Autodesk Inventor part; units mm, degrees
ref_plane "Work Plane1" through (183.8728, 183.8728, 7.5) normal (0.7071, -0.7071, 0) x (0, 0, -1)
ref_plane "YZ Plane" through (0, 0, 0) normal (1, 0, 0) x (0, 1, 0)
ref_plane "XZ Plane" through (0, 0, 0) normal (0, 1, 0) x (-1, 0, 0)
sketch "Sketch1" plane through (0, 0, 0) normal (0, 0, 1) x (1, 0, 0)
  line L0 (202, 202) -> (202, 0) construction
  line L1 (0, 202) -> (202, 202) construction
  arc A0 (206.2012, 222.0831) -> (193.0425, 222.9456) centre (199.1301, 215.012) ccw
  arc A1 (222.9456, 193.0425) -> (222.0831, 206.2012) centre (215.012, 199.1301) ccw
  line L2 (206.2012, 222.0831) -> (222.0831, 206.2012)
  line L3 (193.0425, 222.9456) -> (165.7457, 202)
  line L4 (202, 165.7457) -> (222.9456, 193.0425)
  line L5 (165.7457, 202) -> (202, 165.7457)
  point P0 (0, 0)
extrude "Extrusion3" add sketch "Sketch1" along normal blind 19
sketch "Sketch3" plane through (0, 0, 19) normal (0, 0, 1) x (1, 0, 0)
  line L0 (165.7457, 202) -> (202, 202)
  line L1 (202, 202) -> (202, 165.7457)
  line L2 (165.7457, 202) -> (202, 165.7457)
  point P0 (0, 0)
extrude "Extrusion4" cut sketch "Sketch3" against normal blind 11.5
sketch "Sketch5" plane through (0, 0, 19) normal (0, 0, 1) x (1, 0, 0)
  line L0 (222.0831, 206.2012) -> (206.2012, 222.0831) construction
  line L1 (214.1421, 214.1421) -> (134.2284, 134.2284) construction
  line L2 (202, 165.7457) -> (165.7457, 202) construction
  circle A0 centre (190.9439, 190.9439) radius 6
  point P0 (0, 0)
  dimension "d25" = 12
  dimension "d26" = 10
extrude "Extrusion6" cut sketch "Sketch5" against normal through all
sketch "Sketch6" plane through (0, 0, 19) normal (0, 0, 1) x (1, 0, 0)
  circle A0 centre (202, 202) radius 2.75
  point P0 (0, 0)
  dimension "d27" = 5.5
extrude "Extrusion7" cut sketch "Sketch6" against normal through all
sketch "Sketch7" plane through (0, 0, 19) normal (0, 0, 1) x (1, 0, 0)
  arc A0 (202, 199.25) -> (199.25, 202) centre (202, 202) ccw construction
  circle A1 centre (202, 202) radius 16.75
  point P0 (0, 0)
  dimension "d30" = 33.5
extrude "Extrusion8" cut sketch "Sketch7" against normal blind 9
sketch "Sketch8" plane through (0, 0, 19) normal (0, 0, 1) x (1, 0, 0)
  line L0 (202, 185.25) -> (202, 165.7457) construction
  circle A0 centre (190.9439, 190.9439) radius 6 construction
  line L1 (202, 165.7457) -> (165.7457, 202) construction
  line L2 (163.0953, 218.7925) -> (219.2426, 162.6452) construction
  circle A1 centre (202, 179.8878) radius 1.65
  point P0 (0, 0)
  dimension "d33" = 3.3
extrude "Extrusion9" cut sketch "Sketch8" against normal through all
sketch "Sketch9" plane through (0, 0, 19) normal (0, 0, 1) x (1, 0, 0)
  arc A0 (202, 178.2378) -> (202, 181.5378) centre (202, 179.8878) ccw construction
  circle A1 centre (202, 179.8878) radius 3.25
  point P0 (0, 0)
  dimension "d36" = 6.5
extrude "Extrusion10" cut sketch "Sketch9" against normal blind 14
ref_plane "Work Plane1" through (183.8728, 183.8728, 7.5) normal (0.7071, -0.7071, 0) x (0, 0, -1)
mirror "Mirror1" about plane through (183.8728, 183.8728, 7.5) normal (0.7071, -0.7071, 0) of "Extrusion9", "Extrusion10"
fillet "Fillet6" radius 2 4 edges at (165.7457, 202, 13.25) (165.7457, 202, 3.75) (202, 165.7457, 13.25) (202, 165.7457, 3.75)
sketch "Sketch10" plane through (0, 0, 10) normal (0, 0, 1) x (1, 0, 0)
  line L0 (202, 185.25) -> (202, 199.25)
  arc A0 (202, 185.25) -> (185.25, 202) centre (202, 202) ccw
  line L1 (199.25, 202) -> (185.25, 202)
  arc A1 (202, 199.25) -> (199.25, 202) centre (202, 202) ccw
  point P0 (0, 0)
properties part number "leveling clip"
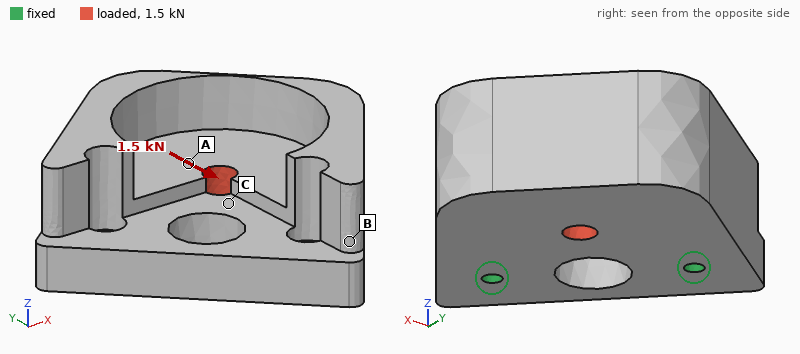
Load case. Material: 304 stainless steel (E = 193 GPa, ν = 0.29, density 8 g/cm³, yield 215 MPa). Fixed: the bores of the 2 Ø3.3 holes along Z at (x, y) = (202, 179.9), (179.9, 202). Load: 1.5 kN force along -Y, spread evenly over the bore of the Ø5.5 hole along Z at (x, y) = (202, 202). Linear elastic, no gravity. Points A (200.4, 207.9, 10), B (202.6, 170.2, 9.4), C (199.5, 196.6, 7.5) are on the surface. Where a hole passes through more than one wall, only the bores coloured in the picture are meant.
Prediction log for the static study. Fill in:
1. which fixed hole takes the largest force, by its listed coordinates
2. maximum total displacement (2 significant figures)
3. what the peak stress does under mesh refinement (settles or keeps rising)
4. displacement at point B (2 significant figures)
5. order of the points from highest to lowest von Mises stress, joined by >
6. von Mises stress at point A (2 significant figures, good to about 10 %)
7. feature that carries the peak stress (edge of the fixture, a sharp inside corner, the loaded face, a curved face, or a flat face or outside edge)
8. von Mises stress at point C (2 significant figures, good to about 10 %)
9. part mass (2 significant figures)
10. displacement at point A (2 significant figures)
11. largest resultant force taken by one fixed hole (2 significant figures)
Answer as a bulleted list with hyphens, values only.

- (202, 179.9)
- 4.0 µm
- keeps rising
- 1.7 µm
- C > A > B
- 6.3 MPa
- edge of the fixture
- 16 MPa
- 170 g
- 2.6 µm
- 1.2 kN
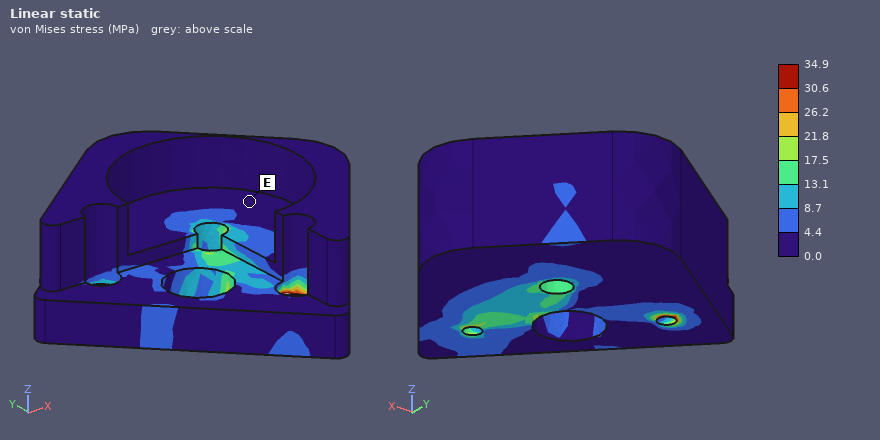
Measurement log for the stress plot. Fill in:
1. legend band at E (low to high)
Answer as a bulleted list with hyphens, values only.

- 0.0 to 4.4 MPa
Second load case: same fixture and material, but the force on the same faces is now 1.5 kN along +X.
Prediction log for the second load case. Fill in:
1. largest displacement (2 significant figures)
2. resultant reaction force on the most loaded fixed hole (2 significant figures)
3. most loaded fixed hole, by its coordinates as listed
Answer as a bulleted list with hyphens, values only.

- 4.0 µm
- 1.2 kN
- (179.9, 202)
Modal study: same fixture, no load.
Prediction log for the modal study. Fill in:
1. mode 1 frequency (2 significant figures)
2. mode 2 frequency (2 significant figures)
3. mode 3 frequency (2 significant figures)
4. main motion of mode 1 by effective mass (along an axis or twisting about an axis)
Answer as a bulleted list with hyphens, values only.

- 3200 Hz
- 7700 Hz
- 11 kHz
- along Z
